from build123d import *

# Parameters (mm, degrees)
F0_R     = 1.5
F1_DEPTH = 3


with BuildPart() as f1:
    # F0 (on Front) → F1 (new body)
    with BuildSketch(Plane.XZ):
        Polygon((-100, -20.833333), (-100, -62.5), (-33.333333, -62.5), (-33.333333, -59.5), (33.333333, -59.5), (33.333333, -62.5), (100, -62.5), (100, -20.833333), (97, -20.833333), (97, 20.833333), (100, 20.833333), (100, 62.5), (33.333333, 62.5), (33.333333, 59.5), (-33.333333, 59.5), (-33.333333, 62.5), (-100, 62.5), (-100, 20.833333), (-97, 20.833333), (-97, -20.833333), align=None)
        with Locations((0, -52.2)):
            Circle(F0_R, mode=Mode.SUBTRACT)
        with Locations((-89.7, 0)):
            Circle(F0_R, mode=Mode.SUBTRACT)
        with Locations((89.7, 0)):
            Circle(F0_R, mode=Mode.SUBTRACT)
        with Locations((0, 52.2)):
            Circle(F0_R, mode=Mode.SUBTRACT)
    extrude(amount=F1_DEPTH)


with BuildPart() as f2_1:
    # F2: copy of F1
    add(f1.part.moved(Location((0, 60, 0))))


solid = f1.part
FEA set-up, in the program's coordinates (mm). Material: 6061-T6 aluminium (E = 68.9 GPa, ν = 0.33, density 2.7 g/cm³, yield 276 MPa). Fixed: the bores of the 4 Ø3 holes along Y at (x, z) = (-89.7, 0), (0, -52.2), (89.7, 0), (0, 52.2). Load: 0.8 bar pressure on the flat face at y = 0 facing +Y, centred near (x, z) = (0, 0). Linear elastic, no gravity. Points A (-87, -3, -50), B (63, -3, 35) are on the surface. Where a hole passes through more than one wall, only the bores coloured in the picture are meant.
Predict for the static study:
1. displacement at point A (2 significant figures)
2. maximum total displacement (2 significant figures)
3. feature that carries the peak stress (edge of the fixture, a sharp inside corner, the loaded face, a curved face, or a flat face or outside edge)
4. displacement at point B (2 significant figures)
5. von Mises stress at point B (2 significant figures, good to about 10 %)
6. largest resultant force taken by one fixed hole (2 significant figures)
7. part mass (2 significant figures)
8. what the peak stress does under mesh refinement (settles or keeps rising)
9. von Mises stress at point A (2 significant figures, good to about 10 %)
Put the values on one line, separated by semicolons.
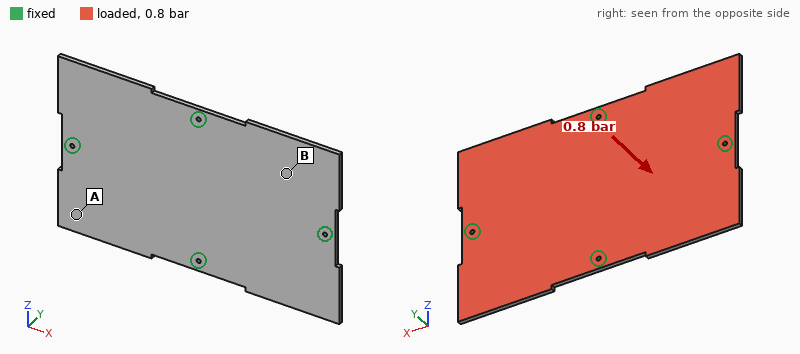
0.45 mm; 0.60 mm; edge of the fixture; 0.30 mm; 32 MPa; 490 N; 200 g; keeps rising; 16 MPa
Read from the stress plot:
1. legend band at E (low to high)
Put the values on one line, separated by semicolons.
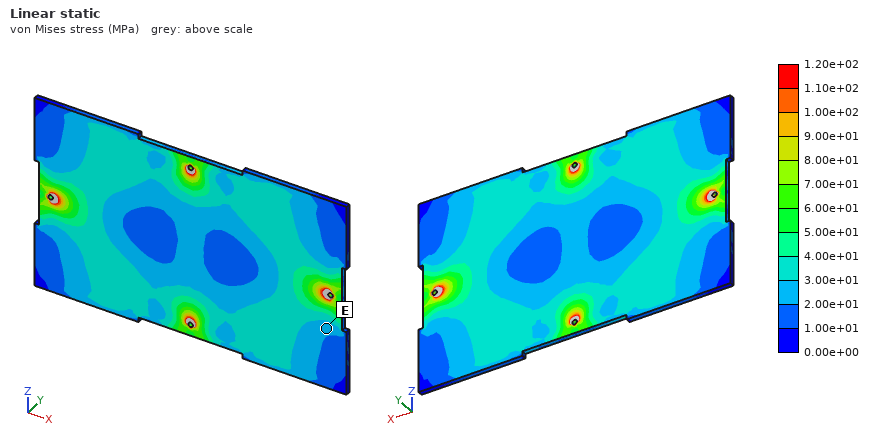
2.00e+01 to 3.00e+01 MPa
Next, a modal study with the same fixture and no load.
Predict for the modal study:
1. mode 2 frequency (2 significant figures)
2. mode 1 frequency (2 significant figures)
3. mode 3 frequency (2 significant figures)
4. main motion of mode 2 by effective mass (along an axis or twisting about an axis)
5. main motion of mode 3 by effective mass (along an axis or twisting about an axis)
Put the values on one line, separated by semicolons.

720 Hz; 690 Hz; 800 Hz; twisting about X; twisting about Z
